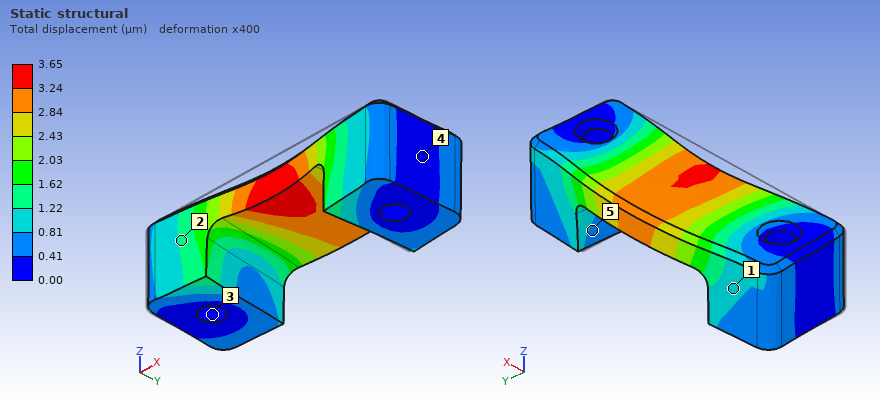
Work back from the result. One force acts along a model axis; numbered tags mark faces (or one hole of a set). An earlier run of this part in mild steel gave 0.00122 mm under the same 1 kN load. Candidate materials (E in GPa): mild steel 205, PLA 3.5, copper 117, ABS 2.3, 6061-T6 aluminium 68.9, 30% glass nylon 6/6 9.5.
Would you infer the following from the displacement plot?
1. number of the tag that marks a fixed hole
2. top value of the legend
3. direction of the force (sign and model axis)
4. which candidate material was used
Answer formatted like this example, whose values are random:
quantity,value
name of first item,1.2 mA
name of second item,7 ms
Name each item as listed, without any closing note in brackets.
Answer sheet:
quantity,value
number of the tag that marks a fixed hole,3
top value of the legend,3.65 µm
direction of the force,+Y
which candidate material was used,6061-T6 aluminium
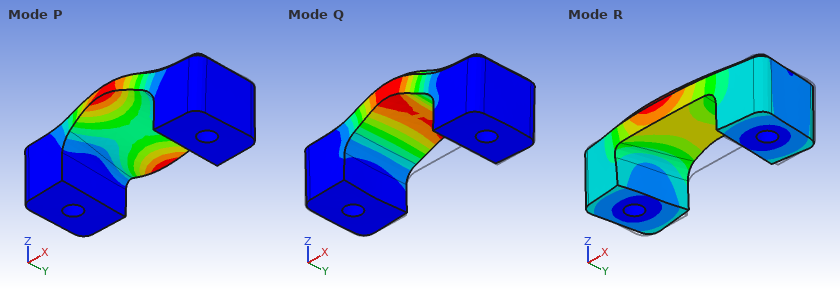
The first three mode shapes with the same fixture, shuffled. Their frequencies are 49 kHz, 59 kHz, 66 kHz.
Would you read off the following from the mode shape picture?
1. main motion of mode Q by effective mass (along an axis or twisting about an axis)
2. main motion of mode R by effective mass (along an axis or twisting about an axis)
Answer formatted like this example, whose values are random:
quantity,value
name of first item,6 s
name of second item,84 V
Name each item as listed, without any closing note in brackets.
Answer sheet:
quantity,value
main motion of mode Q by effective mass,along Z
main motion of mode R by effective mass,along Y
